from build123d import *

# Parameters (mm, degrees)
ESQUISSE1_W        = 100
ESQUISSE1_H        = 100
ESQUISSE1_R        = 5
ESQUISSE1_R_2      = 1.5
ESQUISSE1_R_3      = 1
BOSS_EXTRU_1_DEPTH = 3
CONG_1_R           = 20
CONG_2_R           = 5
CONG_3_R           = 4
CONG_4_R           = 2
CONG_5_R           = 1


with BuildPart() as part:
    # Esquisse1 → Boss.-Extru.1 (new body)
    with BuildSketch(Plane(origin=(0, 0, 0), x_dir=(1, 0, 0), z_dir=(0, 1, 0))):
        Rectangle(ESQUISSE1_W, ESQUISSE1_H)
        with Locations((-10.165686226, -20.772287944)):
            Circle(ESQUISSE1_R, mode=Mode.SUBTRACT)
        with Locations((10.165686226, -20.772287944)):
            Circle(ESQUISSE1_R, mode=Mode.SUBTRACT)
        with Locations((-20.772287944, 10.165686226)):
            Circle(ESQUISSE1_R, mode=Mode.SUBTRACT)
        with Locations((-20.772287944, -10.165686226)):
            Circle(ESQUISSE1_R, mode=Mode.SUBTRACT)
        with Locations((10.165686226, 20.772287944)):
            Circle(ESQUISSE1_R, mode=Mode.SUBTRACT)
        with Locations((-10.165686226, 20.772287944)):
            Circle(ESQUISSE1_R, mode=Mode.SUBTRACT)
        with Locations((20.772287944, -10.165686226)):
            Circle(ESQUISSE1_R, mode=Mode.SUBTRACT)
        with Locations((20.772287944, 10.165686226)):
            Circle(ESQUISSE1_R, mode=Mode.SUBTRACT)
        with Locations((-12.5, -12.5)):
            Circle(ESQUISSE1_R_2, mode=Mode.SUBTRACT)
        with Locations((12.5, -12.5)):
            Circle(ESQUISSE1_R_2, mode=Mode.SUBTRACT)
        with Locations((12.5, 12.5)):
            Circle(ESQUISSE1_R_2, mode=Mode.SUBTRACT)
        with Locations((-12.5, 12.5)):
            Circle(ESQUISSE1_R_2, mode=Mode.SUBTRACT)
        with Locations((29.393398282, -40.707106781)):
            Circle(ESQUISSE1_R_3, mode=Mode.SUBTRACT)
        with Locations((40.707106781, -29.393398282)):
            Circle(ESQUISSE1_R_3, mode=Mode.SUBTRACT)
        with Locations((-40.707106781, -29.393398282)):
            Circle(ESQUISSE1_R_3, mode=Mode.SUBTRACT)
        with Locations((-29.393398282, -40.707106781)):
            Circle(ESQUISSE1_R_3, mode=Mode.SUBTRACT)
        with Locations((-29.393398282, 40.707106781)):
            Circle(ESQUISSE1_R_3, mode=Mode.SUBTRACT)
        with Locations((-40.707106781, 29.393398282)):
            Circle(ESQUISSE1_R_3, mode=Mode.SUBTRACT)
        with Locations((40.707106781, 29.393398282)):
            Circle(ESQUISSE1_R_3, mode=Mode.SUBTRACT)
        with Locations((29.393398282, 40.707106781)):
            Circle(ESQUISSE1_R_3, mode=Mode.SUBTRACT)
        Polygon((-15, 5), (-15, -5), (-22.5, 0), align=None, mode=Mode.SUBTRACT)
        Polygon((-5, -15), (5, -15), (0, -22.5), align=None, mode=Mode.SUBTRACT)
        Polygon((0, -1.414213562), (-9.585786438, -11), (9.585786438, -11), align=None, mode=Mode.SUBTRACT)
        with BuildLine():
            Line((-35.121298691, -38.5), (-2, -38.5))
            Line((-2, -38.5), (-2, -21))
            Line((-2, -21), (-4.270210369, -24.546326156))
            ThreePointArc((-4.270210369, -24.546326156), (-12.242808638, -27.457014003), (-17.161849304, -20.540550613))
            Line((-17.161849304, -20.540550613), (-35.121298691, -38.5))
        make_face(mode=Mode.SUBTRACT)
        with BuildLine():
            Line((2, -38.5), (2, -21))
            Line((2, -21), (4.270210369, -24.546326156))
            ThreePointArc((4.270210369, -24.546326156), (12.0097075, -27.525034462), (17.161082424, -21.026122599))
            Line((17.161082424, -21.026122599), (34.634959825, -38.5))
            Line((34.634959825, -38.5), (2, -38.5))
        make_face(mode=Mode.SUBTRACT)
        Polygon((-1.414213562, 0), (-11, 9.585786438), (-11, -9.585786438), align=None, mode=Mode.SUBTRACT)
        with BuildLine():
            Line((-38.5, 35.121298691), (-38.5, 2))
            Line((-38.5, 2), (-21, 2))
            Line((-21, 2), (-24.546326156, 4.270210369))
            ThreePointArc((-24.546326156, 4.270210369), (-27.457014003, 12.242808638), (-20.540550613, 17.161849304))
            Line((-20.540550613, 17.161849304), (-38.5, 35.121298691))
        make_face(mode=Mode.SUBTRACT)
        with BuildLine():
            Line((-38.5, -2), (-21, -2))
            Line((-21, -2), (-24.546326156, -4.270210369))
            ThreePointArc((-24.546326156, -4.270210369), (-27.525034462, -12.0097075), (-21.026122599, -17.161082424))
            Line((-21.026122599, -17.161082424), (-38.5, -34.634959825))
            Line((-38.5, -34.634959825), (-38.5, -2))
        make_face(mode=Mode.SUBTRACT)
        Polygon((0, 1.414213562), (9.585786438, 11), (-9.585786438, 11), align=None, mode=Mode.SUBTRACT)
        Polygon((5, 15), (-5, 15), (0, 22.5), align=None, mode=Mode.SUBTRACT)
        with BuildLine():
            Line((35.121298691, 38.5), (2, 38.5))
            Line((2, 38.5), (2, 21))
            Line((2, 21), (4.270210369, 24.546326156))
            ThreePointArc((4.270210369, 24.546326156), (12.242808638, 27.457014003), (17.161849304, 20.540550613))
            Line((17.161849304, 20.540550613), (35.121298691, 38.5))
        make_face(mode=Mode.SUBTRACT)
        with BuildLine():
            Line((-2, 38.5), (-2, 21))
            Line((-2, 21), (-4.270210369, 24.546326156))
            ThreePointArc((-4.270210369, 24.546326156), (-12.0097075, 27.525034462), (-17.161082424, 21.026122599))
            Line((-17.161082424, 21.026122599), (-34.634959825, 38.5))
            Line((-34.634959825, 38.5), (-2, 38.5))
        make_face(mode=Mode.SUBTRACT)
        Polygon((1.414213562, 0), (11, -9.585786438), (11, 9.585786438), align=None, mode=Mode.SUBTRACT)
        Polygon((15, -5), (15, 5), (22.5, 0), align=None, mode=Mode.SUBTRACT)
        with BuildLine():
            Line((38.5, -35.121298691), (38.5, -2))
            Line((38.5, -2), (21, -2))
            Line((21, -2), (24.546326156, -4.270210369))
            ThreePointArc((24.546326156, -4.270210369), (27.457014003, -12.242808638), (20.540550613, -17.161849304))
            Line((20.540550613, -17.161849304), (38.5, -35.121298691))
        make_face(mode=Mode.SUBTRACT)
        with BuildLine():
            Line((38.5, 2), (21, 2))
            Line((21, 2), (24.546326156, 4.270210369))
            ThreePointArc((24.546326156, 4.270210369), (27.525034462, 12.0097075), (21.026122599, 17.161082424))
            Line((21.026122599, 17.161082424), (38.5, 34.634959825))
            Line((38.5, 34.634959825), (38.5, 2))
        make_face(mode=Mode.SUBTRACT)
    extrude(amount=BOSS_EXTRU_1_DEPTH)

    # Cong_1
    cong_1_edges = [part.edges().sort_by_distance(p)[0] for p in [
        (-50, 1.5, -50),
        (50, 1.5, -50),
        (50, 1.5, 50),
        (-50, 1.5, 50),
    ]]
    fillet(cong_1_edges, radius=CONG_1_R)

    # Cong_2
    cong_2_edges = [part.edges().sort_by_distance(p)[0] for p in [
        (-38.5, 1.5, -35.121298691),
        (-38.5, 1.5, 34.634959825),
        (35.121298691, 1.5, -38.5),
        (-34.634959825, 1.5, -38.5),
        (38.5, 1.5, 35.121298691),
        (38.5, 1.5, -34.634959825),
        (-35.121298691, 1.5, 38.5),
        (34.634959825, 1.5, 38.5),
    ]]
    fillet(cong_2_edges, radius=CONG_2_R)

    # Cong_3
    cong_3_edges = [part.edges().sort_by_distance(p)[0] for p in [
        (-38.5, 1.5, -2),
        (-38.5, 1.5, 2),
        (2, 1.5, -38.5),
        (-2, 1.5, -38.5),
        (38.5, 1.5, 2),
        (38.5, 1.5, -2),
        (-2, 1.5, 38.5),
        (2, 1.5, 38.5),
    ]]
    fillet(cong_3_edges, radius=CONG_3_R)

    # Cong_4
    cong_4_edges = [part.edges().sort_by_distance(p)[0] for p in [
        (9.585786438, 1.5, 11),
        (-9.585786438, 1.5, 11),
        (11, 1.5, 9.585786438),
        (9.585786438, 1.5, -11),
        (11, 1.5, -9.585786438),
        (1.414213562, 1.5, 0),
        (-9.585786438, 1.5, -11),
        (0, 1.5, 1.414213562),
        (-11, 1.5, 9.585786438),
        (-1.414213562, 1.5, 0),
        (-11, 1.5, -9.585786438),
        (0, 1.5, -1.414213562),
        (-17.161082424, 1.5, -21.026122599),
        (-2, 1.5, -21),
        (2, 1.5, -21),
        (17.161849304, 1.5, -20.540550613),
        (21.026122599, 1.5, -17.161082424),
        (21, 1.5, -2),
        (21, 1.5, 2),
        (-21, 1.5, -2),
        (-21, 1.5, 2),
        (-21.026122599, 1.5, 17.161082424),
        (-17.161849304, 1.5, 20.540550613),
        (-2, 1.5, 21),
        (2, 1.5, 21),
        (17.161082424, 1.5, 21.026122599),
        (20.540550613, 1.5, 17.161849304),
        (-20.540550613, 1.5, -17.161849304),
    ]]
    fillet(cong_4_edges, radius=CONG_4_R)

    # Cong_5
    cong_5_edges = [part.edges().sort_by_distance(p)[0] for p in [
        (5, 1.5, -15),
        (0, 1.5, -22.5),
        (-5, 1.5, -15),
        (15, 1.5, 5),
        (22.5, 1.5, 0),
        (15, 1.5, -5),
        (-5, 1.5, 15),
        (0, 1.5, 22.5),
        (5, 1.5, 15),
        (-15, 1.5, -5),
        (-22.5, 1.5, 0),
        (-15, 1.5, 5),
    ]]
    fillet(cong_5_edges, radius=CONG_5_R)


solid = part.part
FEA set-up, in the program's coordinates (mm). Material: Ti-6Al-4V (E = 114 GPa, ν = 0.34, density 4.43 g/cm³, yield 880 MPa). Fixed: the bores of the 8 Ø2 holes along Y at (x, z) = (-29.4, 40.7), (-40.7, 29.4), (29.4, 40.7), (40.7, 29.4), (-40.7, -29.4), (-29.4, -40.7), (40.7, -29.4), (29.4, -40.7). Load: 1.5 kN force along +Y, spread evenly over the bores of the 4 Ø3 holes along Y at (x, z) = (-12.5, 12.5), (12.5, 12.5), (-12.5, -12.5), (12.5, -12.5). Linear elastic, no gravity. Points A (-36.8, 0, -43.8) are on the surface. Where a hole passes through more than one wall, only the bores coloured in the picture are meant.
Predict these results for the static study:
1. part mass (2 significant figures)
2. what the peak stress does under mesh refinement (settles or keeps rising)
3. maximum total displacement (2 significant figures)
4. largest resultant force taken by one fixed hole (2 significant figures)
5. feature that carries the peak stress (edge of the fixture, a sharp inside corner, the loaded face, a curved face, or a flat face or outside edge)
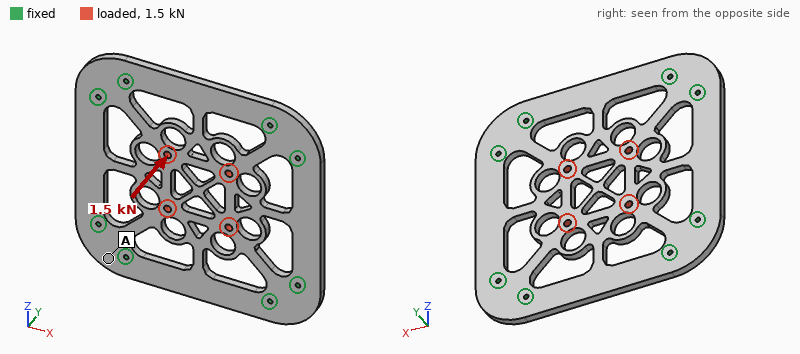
81 g
keeps rising
0.71 mm
190 N
edge of the fixture
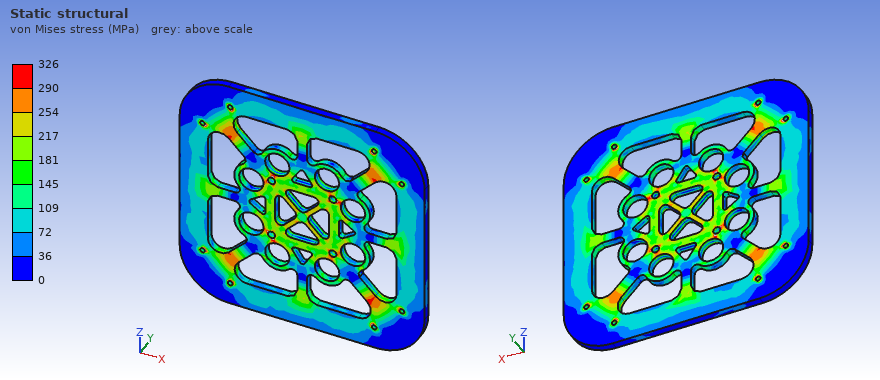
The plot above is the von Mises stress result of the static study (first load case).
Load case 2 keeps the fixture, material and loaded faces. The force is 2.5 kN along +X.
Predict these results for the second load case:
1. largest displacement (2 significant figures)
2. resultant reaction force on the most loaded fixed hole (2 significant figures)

16 µm
530 N
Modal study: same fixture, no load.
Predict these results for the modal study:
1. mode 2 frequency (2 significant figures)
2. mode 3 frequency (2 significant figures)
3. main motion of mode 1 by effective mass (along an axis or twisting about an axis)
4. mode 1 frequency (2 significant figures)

3700 Hz
3700 Hz
along Y
2000 Hz
